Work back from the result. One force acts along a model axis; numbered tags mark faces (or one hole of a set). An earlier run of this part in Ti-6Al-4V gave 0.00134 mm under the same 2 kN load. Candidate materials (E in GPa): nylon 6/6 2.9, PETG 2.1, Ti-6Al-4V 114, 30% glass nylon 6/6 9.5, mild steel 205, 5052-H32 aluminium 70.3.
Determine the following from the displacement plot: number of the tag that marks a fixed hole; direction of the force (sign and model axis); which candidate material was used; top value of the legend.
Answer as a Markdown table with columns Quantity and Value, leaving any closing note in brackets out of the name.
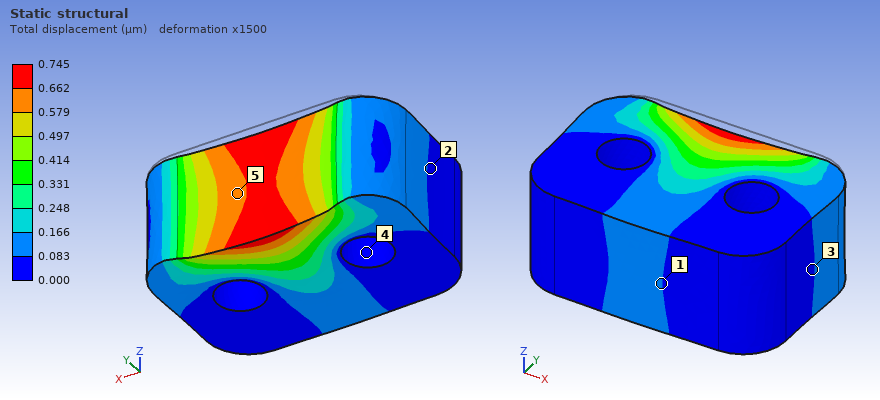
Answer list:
| Quantity | Value |
|---|---|
| number of the tag that marks a fixed hole | 4 |
| direction of the force | -Y |
| which candidate material was used | mild steel |
| top value of the legend | 0.745 µm |
